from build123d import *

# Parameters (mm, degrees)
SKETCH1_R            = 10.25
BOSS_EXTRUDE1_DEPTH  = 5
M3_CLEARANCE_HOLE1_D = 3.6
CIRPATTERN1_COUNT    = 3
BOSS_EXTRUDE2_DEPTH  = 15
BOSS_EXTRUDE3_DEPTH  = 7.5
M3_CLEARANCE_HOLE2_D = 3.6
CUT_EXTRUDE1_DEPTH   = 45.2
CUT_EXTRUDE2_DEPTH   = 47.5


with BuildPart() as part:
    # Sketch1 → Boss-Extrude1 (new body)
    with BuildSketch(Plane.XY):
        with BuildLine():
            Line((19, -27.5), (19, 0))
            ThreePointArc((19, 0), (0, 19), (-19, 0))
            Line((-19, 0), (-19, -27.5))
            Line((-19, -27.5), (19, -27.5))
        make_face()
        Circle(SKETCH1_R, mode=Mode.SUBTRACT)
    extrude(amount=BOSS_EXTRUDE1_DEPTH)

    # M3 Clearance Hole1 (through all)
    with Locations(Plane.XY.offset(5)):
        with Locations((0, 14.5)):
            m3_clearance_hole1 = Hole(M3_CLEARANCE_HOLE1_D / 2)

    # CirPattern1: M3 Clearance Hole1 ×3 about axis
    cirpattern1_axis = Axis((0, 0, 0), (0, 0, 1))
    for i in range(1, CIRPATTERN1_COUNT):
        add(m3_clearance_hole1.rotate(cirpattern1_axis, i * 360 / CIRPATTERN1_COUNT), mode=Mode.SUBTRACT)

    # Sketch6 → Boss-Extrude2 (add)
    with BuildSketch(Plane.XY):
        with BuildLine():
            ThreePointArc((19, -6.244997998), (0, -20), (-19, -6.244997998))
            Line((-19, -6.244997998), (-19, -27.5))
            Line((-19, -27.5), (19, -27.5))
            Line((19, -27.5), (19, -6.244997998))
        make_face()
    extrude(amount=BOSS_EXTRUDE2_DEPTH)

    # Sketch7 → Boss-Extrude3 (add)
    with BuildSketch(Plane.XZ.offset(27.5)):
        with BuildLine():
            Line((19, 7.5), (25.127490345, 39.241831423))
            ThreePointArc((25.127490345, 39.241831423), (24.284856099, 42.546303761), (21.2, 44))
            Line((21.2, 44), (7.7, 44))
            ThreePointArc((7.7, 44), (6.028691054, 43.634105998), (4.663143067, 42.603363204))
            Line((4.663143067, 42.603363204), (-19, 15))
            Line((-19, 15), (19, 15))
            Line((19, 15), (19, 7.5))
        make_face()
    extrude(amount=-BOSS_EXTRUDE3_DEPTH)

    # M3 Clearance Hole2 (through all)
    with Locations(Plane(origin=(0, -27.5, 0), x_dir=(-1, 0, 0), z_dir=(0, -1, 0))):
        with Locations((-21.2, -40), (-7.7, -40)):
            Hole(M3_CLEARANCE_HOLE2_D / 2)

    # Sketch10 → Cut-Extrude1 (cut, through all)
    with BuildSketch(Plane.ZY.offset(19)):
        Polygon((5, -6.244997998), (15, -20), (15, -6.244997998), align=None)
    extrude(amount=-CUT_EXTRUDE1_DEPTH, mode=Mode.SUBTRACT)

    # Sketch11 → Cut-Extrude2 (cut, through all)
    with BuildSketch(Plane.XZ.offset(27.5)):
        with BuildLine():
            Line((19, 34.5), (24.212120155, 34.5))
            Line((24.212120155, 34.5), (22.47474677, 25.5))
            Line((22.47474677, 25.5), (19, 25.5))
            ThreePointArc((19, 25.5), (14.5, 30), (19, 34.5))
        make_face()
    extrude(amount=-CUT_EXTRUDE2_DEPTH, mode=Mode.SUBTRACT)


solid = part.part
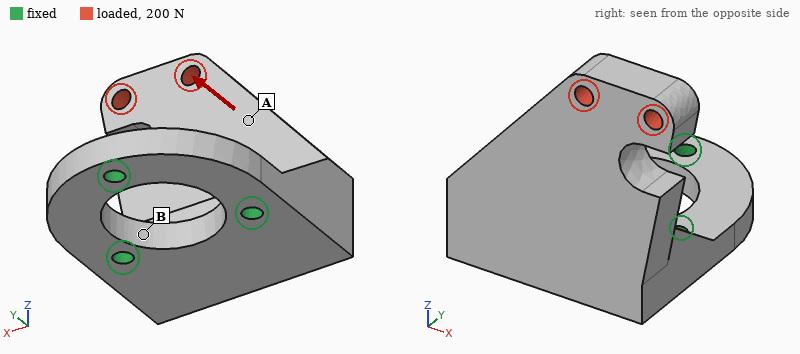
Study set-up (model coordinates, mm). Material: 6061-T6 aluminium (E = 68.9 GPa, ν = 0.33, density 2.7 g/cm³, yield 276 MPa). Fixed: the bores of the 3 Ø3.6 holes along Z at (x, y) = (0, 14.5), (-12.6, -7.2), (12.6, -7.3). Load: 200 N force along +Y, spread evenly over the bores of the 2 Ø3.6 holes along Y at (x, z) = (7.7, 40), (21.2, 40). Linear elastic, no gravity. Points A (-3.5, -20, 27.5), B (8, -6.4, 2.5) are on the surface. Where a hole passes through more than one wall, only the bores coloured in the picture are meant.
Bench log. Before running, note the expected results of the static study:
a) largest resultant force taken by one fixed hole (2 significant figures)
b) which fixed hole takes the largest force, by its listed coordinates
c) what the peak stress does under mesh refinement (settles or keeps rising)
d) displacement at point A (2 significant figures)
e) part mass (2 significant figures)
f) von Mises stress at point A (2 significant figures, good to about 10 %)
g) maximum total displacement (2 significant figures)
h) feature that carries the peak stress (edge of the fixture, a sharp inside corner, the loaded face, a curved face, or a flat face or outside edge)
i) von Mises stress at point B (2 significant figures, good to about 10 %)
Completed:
190 N
(12.6, -7.3)
keeps rising
0.081 mm
43 g
13 MPa
0.18 mm
edge of the fixture
40 MPa
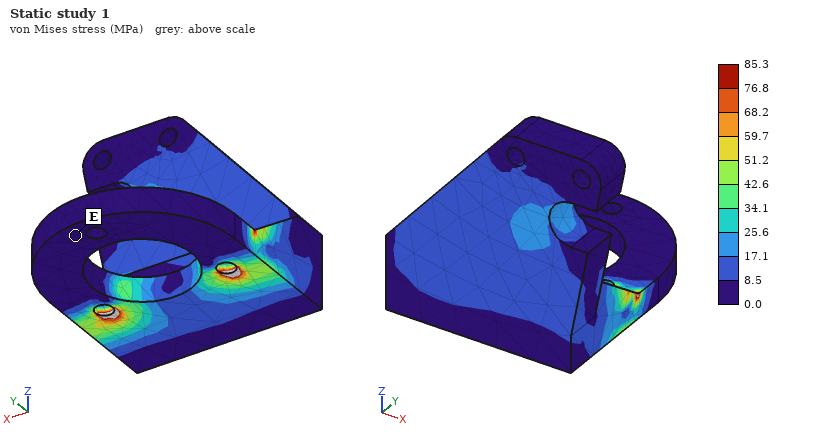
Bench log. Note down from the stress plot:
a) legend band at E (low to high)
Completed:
0.0 to 8.5 MPa
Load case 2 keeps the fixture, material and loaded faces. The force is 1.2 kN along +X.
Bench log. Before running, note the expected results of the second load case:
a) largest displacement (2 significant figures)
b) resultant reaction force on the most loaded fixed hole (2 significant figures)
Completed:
0.17 mm
1.7 kN
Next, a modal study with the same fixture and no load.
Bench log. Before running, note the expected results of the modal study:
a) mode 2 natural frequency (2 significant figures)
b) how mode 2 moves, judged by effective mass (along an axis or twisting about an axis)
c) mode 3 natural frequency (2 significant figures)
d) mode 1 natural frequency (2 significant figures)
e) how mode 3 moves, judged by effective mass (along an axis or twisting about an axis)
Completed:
5100 Hz
along X
7800 Hz
2000 Hz
along Z
